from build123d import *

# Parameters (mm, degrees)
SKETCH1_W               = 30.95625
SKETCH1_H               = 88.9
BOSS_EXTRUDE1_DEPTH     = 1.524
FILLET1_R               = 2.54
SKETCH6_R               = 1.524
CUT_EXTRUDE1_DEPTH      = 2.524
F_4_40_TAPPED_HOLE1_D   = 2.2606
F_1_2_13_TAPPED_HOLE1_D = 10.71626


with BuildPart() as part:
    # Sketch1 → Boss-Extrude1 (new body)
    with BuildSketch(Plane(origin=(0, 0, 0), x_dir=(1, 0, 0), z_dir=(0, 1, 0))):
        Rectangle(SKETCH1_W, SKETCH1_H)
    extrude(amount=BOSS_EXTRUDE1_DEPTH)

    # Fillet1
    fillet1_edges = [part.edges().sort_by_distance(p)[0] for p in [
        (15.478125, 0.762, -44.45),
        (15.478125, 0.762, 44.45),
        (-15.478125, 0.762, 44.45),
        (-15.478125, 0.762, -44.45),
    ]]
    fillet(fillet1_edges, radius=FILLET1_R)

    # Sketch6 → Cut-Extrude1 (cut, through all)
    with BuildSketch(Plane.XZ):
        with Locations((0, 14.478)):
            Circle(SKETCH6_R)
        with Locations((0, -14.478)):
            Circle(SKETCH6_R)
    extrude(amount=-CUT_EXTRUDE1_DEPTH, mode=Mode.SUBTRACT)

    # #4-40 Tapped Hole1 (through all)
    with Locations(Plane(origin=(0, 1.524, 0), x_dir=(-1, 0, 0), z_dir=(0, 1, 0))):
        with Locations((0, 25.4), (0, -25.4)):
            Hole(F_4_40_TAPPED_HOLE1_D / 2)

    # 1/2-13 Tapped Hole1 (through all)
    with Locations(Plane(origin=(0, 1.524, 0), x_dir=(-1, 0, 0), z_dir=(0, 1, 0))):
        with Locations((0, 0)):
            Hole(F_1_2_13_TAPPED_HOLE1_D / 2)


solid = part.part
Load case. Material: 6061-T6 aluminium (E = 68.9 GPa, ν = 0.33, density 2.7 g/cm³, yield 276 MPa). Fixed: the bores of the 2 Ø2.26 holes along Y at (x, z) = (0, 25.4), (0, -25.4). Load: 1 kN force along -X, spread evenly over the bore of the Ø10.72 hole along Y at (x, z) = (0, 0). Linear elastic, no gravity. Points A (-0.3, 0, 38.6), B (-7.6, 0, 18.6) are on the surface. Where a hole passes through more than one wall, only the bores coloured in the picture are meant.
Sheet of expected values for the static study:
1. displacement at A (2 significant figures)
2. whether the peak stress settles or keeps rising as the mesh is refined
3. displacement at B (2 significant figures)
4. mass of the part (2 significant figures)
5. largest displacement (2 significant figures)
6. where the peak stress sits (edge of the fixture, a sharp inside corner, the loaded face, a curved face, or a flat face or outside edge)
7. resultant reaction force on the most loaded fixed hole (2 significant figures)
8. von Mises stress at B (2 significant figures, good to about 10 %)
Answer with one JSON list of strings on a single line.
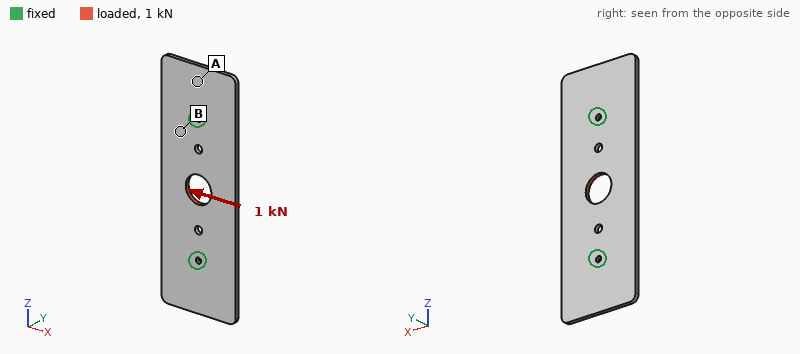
["6.1 µm", "keeps rising", "9.2 µm", "11 g", "23 µm", "edge of the fixture", "500 N", "22 MPa"]
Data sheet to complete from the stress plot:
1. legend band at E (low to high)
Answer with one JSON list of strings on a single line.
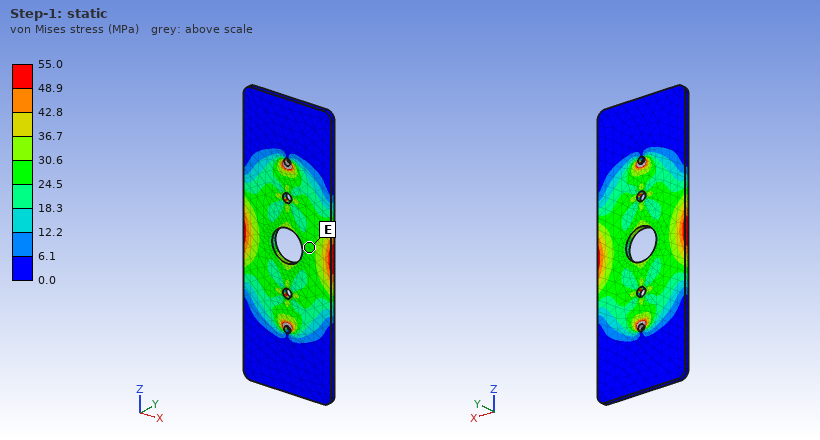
["24.5 to 30.6 MPa"]
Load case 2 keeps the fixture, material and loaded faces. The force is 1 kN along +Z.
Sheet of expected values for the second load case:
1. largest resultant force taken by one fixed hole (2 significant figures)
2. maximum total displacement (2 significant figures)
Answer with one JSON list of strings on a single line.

["500 N", "7.6 µm"]
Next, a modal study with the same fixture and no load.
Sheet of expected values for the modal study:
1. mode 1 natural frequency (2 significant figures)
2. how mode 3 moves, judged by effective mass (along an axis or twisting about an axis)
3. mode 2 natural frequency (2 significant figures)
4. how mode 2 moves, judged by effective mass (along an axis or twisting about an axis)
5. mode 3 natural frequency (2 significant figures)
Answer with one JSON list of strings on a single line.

["2300 Hz", "twisting about X", "2500 Hz", "twisting about Z", "2900 Hz"]
